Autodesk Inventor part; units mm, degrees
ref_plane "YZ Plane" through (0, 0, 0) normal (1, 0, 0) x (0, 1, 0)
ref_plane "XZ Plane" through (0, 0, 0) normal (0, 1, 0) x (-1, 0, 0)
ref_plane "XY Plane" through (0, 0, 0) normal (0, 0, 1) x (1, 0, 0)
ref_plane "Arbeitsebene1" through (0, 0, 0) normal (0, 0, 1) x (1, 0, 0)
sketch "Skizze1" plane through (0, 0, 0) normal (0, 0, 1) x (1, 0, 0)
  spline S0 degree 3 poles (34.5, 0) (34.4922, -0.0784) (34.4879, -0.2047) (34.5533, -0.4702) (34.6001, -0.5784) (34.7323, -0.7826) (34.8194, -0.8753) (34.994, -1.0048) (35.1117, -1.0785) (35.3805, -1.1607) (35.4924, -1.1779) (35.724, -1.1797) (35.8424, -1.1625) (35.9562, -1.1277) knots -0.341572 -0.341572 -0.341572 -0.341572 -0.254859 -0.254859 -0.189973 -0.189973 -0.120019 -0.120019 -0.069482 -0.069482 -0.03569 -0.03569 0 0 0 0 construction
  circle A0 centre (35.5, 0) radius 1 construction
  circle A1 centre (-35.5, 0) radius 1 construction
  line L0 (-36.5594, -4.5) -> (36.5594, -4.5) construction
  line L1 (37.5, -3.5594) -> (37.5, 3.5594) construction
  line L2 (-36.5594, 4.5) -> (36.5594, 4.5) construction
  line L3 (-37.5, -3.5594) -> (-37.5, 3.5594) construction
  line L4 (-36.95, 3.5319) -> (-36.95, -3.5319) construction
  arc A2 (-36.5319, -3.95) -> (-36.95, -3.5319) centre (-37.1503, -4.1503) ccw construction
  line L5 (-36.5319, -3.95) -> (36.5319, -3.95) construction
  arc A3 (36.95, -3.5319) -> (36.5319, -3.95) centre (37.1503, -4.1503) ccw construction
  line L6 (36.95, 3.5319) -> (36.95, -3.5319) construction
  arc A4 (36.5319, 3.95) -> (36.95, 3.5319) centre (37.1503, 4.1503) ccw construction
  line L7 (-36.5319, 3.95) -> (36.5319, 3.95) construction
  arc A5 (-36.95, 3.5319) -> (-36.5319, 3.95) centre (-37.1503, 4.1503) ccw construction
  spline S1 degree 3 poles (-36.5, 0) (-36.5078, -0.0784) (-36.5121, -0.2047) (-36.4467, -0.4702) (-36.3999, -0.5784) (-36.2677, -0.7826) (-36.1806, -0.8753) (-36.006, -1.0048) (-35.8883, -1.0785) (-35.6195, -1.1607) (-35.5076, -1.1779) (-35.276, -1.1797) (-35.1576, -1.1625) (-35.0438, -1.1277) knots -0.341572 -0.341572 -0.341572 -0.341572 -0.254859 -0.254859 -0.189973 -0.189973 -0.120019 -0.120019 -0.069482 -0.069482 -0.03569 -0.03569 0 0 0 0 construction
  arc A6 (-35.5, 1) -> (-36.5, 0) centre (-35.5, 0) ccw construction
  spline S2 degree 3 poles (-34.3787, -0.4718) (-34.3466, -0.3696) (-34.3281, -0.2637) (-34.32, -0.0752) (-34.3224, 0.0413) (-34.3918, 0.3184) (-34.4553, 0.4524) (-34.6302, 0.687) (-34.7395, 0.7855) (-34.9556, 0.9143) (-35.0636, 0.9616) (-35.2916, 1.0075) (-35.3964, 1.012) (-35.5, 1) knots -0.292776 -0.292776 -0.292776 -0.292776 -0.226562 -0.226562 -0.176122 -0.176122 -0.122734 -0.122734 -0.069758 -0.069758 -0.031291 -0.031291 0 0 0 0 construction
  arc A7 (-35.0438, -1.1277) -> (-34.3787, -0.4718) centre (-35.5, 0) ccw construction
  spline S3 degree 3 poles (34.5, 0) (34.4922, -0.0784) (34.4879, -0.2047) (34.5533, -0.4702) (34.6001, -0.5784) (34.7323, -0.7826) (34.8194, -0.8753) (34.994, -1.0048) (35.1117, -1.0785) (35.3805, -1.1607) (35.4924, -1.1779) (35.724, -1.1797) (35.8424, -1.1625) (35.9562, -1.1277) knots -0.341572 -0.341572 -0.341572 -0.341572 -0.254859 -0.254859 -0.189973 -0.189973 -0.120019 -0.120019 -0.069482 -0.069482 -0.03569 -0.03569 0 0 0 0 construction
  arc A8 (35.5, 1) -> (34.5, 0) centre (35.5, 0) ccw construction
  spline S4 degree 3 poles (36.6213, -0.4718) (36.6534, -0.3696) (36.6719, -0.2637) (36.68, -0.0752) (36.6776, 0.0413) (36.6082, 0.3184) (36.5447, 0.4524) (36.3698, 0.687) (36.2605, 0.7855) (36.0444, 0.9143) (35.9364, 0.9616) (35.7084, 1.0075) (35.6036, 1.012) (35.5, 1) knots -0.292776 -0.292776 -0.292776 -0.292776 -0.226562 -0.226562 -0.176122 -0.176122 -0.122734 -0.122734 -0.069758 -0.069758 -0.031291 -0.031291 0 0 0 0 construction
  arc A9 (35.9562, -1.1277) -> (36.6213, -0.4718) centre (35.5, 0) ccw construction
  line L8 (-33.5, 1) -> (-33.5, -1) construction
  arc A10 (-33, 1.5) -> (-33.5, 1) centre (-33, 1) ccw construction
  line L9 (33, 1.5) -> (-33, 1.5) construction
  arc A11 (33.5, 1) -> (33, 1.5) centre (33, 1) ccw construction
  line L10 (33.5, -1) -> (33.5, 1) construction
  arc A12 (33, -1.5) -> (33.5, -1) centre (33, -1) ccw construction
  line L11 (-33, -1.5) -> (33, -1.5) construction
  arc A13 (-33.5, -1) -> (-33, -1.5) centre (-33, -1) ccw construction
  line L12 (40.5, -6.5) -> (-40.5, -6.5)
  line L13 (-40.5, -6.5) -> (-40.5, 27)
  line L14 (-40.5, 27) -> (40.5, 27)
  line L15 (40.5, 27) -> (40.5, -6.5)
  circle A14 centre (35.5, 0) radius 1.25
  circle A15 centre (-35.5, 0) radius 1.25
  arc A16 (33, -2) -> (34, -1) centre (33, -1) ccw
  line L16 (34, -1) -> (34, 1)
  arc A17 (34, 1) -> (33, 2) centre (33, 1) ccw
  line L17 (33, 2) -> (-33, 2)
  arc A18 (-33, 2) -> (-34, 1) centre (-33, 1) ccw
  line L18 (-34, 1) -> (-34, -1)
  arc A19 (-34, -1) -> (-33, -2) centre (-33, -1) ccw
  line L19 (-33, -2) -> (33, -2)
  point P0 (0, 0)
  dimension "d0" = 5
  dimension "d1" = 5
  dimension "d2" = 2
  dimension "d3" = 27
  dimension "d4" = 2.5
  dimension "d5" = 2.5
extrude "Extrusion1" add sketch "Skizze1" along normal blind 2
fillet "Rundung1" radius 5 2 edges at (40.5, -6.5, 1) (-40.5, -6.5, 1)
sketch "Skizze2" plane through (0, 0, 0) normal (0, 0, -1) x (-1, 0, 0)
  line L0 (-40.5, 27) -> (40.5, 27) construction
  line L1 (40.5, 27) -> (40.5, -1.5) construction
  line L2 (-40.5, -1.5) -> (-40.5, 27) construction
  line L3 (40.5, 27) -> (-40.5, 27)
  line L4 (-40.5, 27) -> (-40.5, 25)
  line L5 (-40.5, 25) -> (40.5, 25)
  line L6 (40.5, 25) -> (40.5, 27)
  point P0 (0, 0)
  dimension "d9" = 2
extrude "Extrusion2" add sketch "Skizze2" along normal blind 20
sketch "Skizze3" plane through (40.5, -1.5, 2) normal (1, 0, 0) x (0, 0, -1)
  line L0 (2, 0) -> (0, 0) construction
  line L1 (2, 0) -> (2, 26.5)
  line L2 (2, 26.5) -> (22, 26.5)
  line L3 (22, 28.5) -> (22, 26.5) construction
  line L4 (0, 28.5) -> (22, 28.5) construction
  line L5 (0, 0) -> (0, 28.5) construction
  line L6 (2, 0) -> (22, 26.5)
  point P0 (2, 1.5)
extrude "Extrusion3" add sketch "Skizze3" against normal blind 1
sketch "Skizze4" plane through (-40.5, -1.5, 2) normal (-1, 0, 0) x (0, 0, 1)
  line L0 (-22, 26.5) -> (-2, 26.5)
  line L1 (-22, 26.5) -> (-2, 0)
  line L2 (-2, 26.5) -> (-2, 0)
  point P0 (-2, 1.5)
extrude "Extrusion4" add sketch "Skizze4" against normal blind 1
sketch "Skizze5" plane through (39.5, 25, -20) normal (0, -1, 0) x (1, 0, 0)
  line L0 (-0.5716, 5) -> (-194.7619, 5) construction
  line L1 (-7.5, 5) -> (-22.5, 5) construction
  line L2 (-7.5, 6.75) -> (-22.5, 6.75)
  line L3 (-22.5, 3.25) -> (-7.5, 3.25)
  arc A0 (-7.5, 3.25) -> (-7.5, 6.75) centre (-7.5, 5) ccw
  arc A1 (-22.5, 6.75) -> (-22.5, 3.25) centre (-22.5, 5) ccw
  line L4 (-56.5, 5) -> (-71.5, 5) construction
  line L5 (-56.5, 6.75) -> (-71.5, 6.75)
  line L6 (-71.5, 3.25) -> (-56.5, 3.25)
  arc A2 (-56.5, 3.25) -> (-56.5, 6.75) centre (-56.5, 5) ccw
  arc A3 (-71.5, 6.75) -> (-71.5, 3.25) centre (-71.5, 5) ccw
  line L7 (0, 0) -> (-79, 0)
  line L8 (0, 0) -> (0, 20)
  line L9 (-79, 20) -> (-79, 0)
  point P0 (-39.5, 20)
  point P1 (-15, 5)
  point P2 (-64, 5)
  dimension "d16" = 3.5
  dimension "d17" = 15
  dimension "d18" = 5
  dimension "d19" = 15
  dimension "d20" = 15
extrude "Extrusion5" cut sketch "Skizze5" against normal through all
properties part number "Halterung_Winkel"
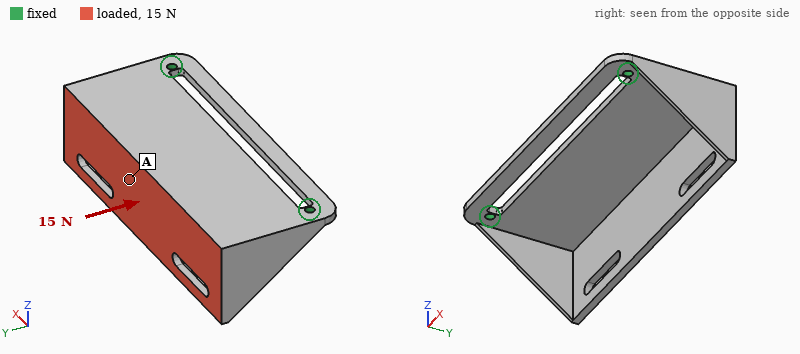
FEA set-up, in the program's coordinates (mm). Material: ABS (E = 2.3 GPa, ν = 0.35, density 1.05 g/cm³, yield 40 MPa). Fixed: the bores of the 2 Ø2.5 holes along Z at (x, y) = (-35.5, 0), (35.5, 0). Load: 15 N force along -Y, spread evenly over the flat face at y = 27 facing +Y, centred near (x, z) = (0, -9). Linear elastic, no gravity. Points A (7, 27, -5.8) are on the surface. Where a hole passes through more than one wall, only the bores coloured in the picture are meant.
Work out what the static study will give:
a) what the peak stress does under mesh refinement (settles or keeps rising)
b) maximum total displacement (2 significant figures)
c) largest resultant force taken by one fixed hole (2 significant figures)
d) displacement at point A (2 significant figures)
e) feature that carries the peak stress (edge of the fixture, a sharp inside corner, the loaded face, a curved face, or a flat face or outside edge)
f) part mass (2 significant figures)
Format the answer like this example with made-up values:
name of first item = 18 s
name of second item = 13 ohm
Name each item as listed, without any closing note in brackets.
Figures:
what the peak stress does under mesh refinement = keeps rising
maximum total displacement = 0.93 mm
largest resultant force taken by one fixed hole = 8.5 N
displacement at point A = 0.59 mm
feature that carries the peak stress = edge of the fixture
part mass = 8.8 g
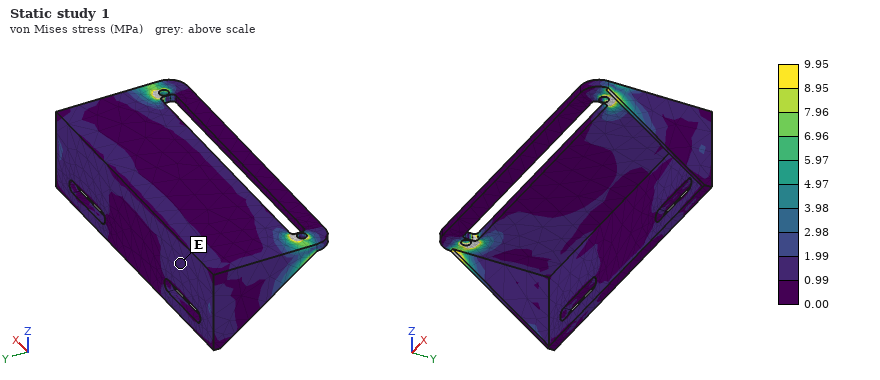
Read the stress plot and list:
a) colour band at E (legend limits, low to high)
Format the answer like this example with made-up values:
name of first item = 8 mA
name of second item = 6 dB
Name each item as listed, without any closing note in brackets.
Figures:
colour band at E = 0.99 to 1.99 MPa
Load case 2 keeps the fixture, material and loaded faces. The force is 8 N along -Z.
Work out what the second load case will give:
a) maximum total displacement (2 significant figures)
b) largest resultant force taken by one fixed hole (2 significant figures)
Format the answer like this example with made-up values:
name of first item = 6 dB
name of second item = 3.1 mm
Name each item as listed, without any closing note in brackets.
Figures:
maximum total displacement = 0.96 mm
largest resultant force taken by one fixed hole = 4.2 N
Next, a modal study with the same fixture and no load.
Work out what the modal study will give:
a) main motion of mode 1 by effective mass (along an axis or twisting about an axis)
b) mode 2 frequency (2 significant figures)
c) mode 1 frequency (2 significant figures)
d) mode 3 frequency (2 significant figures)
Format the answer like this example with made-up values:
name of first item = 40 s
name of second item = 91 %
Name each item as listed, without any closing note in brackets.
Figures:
main motion of mode 1 by effective mass = along Z
mode 2 frequency = 450 Hz
mode 1 frequency = 230 Hz
mode 3 frequency = 570 Hz
